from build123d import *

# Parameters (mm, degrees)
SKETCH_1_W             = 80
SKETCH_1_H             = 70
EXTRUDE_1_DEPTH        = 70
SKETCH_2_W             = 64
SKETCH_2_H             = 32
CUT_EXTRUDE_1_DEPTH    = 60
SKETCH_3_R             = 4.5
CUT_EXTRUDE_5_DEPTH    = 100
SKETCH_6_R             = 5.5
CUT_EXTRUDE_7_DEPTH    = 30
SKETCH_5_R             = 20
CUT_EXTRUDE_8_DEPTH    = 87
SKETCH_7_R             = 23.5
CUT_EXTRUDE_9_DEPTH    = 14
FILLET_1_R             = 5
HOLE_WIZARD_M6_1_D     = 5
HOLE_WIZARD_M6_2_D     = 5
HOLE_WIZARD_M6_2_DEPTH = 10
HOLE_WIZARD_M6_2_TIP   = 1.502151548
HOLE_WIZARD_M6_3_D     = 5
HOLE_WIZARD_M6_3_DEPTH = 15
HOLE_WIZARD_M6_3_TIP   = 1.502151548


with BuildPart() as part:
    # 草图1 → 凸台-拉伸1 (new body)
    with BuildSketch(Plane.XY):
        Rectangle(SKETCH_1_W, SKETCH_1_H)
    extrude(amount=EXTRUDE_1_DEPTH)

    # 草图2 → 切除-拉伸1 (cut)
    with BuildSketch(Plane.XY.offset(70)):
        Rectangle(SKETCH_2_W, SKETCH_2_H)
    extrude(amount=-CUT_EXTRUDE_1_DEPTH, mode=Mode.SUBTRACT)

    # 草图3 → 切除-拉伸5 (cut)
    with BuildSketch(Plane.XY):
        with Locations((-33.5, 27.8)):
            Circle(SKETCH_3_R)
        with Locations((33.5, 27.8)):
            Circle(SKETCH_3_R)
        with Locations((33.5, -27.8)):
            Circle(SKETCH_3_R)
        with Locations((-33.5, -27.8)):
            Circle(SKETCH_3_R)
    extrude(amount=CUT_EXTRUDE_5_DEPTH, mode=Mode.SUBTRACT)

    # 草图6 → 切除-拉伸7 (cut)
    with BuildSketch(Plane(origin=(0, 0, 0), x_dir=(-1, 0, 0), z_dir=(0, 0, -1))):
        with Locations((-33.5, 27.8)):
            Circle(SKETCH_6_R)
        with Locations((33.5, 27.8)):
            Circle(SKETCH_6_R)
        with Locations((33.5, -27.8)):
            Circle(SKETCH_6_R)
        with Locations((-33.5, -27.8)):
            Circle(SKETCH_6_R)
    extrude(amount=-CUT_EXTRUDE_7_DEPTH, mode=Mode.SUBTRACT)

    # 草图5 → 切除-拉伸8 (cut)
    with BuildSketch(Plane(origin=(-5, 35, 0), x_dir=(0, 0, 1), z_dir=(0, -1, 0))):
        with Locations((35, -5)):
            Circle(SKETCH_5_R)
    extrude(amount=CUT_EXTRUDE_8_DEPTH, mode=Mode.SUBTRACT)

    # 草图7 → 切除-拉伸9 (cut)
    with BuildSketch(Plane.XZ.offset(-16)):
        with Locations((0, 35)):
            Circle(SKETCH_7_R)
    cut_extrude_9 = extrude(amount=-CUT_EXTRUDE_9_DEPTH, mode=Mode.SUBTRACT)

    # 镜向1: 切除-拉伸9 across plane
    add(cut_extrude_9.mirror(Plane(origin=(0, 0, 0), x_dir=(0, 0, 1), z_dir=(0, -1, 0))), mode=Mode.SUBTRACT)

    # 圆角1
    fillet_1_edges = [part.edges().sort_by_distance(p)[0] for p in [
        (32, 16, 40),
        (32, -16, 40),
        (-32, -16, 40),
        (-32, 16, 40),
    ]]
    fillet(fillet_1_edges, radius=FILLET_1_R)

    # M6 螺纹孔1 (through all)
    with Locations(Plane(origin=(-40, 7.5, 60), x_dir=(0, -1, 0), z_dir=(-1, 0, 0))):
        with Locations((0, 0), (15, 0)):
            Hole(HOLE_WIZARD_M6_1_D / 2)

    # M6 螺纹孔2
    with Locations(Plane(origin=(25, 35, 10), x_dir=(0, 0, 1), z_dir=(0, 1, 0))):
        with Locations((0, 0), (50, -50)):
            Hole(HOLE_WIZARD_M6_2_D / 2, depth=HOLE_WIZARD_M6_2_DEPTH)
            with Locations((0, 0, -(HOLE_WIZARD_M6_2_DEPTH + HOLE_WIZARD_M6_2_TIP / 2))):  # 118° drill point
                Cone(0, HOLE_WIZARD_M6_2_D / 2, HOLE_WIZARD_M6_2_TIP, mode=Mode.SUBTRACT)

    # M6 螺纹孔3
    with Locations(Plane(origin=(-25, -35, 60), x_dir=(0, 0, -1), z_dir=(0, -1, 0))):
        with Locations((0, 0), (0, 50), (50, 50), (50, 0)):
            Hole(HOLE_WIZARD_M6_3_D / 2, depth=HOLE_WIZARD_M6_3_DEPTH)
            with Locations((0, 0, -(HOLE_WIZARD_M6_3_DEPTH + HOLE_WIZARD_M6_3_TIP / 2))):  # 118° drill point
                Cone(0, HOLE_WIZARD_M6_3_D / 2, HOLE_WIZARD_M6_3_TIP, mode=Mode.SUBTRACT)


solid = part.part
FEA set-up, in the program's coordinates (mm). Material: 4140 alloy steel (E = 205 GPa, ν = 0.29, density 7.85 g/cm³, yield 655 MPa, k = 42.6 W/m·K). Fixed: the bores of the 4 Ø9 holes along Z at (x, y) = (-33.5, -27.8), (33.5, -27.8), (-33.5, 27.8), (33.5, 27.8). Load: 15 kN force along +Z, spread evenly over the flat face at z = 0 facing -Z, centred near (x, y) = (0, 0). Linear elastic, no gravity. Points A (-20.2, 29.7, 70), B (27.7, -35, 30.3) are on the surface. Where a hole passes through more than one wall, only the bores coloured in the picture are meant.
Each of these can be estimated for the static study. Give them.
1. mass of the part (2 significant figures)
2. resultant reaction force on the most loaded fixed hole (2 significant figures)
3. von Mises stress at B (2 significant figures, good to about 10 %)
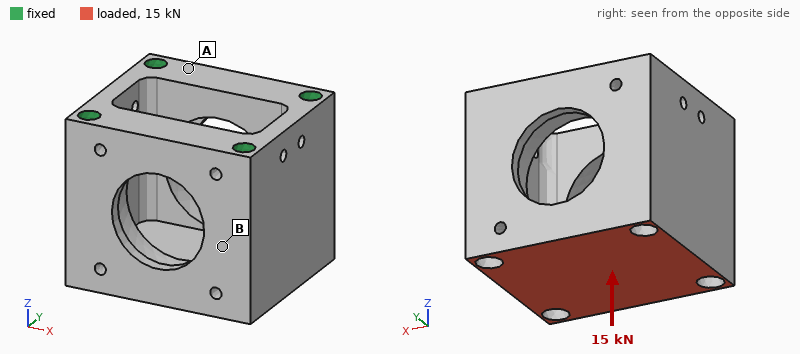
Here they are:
1.5 kg
4.1 kN
14 MPa
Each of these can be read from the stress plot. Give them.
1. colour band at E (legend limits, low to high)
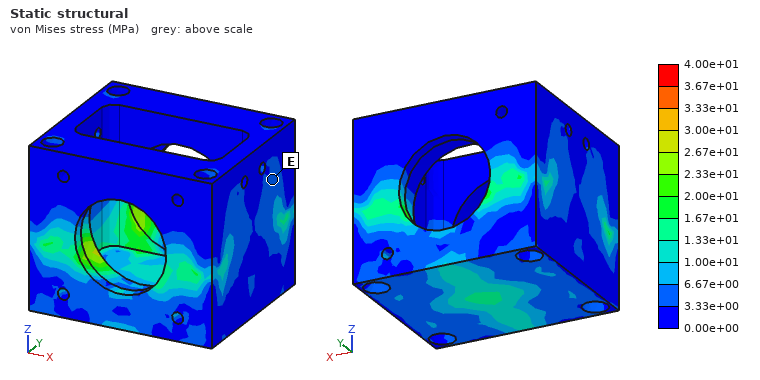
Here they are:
3.33e+00 to 6.67e+00 MPa
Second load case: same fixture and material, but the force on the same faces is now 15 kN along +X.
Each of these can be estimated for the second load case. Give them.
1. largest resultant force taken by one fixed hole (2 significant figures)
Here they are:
4.8 kN
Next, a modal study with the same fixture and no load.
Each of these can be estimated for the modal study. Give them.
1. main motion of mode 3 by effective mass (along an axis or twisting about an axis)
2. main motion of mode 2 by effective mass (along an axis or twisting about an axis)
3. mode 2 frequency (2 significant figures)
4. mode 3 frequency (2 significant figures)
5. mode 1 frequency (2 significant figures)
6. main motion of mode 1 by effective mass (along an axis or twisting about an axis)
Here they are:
twisting about Z
along Y
10 kHz
14 kHz
8600 Hz
along X
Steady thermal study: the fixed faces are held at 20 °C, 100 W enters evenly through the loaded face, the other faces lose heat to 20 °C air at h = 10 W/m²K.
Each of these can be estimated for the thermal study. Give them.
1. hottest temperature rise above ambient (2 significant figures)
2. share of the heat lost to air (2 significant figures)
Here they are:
53 K
6.7 %
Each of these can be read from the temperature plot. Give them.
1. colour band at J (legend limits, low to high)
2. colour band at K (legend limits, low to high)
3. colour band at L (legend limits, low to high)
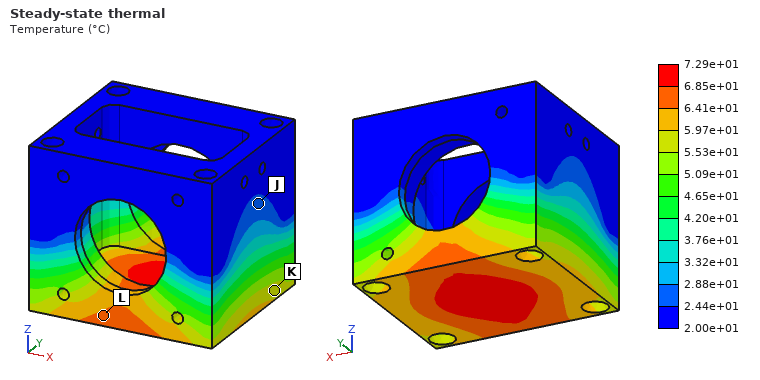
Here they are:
2.44e+01 to 2.88e+01 °C
5.53e+01 to 5.97e+01 °C
6.41e+01 to 6.85e+01 °C
